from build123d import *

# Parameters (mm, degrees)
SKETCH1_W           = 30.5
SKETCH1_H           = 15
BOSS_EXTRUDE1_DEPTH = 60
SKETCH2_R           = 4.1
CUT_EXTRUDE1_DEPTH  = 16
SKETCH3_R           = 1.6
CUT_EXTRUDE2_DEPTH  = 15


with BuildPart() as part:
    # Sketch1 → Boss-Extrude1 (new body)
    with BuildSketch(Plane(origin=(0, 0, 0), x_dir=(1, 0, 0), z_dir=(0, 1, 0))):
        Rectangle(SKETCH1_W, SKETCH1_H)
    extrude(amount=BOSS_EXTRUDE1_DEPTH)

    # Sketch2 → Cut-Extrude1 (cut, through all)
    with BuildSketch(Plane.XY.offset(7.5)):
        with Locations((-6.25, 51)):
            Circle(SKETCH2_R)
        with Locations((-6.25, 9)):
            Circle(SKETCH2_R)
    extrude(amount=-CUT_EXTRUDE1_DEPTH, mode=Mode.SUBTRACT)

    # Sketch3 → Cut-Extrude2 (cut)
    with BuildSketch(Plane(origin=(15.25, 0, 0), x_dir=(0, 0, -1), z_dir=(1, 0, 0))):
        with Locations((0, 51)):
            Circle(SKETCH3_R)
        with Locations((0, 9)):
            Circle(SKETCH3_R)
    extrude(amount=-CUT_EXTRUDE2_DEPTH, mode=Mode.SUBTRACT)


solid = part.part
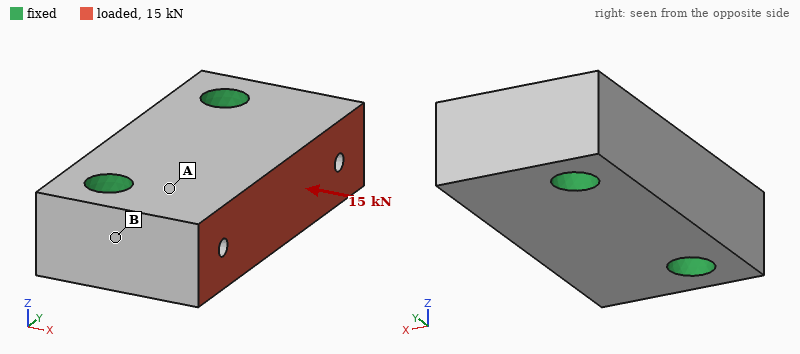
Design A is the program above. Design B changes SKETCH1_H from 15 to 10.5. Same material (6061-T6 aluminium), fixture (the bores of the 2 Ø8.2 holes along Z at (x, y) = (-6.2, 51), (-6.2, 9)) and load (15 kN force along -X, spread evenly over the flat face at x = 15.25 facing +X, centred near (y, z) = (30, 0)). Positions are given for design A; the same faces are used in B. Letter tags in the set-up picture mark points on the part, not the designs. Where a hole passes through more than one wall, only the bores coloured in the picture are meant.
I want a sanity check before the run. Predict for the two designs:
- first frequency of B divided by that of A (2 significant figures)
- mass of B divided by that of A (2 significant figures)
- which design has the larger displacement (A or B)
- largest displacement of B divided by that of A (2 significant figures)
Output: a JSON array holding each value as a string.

["0.82", "0.70", "B", "1.4"]
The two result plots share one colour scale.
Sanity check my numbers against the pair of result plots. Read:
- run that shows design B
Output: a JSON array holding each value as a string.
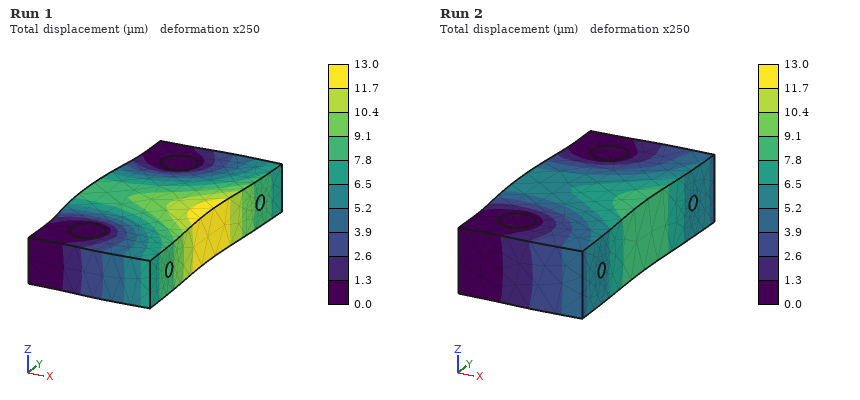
["Run 1"]
